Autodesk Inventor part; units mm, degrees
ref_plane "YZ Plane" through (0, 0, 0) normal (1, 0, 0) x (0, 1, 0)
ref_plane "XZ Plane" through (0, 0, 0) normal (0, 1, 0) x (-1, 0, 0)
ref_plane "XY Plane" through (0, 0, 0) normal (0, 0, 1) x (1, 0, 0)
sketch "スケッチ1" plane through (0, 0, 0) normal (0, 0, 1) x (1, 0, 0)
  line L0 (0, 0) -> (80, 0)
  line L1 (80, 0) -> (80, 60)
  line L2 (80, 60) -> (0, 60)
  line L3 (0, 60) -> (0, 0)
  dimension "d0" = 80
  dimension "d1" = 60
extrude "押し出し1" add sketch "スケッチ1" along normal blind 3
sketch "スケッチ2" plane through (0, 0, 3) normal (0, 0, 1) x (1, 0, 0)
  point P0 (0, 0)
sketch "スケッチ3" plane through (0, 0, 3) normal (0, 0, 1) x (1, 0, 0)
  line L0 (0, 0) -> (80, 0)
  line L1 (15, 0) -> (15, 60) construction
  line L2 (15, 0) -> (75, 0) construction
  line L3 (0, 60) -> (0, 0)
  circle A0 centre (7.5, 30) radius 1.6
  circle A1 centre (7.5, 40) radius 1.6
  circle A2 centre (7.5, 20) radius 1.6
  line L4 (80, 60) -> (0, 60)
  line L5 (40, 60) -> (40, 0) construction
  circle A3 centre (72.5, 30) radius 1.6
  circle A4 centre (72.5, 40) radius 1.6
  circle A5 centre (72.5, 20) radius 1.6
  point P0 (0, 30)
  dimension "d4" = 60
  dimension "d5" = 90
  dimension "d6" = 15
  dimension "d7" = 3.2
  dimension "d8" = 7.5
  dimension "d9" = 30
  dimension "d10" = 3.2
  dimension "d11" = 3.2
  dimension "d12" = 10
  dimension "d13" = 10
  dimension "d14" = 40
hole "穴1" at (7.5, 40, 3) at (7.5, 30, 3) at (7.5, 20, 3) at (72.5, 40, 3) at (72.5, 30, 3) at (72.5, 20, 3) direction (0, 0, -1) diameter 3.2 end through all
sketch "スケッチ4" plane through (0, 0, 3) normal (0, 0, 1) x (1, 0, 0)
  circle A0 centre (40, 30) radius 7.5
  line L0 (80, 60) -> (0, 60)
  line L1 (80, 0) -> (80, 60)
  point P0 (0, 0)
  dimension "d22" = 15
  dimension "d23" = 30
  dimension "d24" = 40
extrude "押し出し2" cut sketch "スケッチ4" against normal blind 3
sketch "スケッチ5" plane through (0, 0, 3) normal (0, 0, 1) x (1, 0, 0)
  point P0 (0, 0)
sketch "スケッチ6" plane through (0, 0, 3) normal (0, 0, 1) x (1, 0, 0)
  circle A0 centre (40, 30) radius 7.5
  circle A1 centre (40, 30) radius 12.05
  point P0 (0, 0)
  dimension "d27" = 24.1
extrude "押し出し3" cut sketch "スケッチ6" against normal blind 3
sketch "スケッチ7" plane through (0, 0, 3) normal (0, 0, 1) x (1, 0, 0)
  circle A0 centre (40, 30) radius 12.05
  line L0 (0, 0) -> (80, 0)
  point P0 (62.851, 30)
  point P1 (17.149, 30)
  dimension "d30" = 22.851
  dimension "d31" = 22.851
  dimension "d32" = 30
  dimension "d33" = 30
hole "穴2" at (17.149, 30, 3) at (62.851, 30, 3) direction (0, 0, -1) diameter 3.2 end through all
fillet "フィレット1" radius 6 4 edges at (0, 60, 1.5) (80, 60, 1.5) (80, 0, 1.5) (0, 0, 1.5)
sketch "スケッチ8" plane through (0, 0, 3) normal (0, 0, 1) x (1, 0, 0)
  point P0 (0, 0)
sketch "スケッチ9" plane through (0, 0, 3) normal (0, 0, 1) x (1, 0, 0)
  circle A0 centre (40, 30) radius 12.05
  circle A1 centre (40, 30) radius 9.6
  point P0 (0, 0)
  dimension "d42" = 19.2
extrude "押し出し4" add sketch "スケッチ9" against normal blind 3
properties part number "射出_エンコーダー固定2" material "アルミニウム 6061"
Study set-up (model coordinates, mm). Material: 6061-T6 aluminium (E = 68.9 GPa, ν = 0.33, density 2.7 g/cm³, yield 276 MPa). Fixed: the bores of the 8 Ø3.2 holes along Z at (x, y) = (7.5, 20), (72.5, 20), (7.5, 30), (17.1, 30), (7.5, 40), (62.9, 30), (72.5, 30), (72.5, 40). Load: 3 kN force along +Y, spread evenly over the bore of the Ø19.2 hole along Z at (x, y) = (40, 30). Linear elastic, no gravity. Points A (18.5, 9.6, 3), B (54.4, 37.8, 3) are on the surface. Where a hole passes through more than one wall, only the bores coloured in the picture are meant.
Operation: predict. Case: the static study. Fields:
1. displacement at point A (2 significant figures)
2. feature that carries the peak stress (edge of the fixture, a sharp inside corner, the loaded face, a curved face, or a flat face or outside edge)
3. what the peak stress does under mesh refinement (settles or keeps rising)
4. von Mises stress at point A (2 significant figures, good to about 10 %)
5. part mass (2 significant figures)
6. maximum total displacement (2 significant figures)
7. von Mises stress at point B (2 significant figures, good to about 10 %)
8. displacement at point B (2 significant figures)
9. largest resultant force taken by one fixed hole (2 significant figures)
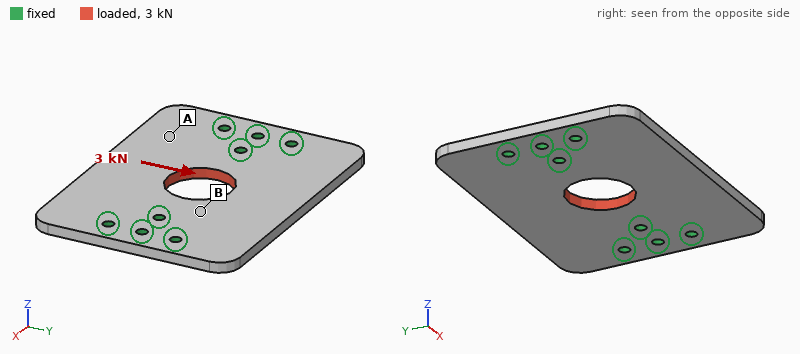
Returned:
4.1 µm
edge of the fixture
keeps rising
8.3 MPa
36 g
11 µm
20 MPa
6.1 µm
1.1 kN
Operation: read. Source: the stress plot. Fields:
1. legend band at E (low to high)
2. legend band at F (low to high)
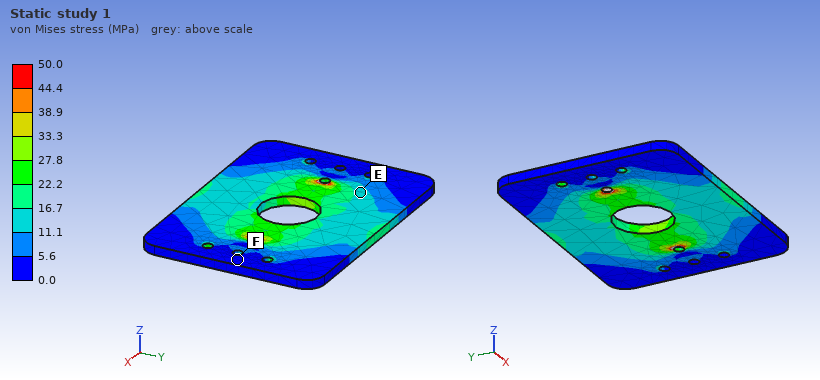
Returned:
11.1 to 16.7 MPa
0.0 to 5.6 MPa
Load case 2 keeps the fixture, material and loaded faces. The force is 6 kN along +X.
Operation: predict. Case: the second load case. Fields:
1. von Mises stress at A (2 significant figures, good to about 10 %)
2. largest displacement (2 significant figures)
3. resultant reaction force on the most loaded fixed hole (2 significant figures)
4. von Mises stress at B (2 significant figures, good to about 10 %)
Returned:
6.6 MPa
13 µm
1.3 kN
33 MPa
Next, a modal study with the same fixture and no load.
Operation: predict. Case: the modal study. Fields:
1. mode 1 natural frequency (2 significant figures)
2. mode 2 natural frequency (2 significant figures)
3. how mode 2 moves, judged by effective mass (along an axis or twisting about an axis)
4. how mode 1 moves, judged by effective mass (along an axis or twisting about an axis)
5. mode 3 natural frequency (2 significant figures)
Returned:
3200 Hz
3400 Hz
along Z
twisting about X
6300 Hz
